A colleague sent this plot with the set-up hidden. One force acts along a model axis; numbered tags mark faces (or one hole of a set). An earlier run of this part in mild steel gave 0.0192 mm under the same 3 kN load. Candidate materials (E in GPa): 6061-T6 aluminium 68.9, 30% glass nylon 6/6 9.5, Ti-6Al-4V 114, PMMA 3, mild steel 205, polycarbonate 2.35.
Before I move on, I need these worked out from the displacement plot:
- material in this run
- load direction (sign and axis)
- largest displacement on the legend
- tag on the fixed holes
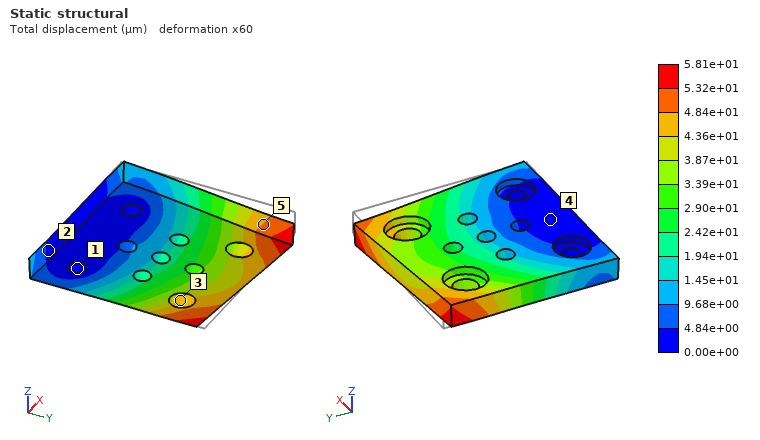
6061-T6 aluminium
-X
5.81e+01 µm
1
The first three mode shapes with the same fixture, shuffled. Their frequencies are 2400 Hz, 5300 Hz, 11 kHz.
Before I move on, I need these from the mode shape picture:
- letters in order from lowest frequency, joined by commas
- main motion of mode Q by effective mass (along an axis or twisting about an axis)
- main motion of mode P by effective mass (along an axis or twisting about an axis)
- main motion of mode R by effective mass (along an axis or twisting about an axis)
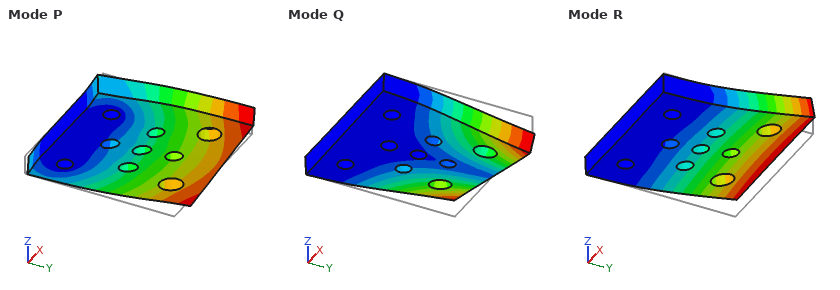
R, Q, P
twisting about Y
along X
along Z
